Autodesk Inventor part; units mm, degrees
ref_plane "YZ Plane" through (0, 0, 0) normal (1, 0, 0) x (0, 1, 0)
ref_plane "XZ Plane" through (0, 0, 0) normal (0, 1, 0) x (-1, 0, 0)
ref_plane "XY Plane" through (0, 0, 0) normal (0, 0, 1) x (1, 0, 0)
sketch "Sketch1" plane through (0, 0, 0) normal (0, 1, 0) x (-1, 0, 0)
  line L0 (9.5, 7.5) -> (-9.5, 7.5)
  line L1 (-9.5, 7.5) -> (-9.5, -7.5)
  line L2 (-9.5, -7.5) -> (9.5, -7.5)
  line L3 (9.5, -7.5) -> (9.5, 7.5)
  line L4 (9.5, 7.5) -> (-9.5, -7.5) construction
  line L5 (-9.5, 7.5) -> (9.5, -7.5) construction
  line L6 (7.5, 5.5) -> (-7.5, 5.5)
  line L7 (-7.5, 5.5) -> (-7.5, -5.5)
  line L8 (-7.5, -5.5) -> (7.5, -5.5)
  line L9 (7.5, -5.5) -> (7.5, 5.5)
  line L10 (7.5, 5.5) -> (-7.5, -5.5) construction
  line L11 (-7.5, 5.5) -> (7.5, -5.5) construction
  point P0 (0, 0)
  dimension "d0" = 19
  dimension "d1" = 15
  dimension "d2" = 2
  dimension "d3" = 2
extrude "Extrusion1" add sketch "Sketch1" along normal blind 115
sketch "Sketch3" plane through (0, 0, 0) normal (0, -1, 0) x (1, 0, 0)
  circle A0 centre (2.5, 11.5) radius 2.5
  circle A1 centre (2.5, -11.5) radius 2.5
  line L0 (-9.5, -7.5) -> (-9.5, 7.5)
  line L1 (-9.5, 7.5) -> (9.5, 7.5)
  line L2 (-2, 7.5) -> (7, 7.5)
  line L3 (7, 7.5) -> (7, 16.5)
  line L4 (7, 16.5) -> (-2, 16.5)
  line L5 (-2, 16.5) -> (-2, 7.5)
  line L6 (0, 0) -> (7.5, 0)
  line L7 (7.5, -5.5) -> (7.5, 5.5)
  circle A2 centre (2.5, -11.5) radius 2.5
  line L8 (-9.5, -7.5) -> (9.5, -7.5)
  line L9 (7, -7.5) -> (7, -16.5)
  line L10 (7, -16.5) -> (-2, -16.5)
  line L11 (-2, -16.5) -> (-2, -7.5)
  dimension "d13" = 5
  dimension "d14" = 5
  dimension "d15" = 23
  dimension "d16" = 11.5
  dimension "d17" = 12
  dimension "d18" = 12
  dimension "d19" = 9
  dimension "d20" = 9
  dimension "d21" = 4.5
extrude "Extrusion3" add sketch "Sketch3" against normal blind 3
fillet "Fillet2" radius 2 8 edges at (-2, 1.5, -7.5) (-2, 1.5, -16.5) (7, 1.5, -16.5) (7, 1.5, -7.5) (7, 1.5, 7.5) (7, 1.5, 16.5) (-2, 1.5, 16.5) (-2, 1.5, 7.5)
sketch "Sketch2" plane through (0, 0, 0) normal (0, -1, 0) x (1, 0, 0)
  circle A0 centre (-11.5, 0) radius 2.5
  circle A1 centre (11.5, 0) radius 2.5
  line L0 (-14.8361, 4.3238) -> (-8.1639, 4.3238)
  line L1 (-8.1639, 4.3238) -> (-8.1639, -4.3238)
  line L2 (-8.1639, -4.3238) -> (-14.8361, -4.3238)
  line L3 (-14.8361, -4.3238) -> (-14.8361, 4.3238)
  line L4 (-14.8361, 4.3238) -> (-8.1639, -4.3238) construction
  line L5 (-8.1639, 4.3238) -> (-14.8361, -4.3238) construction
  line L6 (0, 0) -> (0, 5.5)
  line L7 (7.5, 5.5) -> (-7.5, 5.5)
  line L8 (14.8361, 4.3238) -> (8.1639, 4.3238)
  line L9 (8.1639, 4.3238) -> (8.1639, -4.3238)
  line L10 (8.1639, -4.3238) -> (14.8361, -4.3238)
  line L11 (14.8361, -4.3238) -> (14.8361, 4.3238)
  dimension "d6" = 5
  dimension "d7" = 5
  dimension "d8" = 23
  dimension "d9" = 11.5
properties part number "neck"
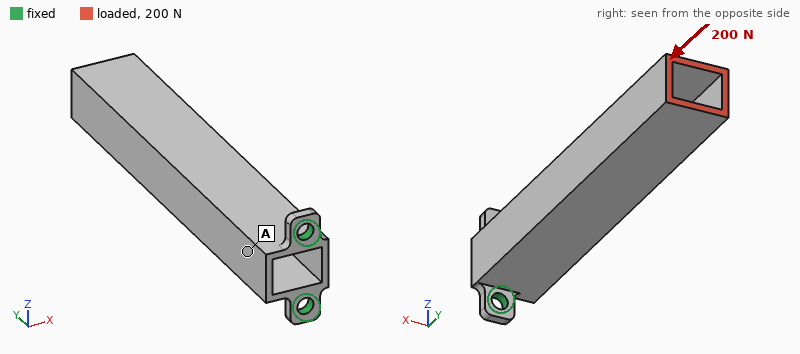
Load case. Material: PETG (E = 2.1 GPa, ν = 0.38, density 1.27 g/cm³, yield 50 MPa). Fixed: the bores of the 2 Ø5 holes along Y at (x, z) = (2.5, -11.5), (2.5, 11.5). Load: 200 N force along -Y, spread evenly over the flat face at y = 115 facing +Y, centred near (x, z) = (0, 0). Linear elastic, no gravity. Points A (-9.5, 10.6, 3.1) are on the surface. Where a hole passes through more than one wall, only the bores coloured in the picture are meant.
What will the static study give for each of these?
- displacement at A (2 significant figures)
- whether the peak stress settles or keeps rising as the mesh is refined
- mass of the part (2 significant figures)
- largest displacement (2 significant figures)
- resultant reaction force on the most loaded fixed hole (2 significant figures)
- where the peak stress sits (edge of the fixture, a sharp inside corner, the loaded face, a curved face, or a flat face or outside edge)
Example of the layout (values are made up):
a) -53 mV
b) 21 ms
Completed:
a) 0.21 mm
b) keeps rising
c) 18 g
d) 1.2 mm
e) 100 N
f) edge of the fixture
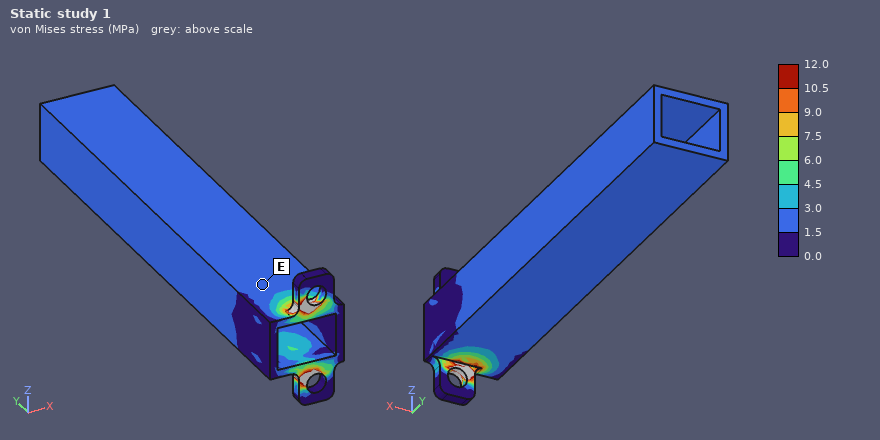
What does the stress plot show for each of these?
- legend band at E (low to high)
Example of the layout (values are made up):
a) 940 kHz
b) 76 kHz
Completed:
a) 1.5 to 3.0 MPa
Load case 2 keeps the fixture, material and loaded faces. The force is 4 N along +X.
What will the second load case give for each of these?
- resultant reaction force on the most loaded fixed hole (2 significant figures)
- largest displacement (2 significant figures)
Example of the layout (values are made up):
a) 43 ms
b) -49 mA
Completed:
a) 2.5 N
b) 1.2 mm
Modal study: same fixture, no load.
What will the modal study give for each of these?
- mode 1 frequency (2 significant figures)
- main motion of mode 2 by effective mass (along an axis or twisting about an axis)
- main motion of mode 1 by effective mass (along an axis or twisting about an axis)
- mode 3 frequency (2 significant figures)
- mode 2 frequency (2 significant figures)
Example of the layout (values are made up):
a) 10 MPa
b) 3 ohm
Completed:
a) 120 Hz
b) along Z
c) along X
d) 1300 Hz
e) 220 Hz
